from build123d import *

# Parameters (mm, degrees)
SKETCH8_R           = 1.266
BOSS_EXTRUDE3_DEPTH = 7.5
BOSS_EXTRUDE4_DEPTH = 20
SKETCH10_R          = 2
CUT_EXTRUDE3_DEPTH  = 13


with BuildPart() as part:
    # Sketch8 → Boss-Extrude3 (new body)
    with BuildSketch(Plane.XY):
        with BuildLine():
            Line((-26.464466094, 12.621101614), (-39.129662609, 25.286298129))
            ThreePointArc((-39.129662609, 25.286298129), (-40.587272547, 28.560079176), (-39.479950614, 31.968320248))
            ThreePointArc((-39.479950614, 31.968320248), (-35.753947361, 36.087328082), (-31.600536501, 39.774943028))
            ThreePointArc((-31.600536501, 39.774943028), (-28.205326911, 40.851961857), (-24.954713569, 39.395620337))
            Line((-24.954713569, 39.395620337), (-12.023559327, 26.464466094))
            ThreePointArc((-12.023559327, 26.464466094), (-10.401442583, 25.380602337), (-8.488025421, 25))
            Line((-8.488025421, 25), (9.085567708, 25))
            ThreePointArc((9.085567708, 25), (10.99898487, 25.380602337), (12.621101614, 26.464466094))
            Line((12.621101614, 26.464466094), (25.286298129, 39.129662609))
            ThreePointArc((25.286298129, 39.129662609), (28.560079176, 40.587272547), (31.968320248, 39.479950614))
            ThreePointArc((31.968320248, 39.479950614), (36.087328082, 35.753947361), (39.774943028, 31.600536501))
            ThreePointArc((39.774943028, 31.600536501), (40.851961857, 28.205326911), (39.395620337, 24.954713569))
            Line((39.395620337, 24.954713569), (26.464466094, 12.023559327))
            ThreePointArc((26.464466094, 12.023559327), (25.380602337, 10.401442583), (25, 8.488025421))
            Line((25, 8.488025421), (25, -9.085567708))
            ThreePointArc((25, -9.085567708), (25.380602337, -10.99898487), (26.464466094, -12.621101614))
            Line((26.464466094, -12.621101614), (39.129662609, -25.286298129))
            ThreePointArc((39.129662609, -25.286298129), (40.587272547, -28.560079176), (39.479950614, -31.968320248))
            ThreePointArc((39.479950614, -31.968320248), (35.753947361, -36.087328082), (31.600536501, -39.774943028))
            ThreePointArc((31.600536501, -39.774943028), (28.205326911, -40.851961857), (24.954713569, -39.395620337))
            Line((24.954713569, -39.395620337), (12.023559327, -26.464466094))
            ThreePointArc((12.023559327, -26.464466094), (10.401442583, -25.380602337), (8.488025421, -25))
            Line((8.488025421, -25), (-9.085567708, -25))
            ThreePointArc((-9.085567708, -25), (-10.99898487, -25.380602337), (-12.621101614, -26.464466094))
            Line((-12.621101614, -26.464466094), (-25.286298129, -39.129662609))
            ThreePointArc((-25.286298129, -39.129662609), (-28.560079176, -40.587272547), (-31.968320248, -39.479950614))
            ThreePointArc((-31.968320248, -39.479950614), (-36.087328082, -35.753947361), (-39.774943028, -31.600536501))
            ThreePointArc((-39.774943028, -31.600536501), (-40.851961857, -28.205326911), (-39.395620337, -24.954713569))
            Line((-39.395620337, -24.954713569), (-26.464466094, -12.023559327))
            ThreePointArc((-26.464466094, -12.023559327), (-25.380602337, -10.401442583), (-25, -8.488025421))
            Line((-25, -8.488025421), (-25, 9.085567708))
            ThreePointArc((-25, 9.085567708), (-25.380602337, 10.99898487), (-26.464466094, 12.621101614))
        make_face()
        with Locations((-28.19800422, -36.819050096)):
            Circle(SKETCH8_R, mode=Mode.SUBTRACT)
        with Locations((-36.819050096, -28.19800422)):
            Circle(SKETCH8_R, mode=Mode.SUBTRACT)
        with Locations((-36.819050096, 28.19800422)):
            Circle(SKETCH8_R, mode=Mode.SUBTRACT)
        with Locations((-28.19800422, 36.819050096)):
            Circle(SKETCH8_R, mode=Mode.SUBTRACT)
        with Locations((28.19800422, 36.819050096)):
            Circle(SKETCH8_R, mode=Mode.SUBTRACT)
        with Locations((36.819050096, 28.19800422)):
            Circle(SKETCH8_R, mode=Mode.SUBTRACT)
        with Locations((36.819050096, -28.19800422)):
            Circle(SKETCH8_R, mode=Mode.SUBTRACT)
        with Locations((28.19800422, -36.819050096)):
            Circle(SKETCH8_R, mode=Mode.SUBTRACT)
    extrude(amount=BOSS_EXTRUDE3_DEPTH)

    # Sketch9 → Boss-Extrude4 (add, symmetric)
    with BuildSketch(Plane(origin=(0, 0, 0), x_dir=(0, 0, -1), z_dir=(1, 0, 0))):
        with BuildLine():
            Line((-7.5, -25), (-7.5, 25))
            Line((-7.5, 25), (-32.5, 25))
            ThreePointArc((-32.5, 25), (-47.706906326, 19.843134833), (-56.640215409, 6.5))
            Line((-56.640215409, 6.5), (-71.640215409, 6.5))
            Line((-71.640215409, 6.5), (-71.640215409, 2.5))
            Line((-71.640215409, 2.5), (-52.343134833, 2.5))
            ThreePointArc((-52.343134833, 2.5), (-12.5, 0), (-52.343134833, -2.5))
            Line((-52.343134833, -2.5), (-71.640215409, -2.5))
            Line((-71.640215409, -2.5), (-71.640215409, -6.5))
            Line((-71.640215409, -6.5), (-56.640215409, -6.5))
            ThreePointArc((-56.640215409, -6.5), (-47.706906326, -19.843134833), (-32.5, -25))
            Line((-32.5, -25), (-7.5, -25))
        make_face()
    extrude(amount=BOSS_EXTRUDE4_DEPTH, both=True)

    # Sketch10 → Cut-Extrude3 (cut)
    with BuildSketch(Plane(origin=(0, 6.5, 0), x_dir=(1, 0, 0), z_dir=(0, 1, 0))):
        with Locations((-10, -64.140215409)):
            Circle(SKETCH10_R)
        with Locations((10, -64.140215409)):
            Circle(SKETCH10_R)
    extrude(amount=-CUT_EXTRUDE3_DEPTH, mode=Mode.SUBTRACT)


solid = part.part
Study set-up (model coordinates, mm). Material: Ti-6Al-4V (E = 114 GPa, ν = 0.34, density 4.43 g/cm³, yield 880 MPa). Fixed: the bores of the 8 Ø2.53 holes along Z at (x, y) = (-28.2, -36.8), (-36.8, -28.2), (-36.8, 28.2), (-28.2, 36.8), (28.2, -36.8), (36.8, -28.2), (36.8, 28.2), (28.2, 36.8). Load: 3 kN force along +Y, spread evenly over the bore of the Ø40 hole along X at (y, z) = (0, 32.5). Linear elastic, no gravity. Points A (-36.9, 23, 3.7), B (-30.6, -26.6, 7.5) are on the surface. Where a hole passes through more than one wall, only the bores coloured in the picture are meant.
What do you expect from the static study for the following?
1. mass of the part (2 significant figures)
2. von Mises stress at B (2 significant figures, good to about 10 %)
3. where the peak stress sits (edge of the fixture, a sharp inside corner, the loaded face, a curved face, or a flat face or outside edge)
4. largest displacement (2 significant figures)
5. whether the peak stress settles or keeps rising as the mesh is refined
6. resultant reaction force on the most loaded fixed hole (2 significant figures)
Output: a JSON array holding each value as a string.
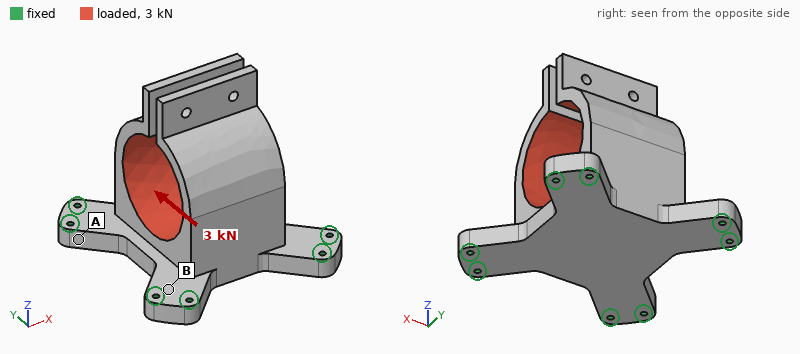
["320 g", "9.9 MPa", "edge of the fixture", "0.20 mm", "keeps rising", "850 N"]
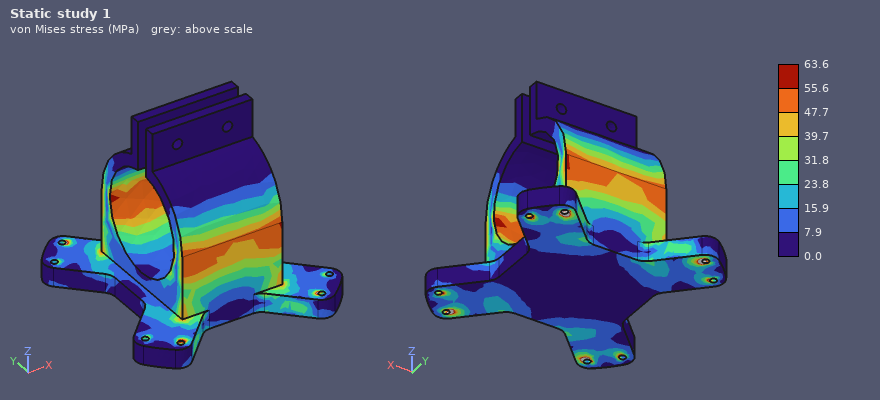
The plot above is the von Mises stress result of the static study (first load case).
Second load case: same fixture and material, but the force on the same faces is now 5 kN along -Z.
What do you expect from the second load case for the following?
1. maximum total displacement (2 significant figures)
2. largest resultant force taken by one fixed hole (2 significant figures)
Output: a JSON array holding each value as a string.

["0.22 mm", "790 N"]
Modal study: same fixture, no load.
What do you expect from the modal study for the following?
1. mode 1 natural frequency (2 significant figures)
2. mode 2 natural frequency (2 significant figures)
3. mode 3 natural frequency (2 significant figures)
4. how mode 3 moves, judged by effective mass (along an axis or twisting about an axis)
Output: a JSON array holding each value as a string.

["1500 Hz", "1500 Hz", "3200 Hz", "along X"]
